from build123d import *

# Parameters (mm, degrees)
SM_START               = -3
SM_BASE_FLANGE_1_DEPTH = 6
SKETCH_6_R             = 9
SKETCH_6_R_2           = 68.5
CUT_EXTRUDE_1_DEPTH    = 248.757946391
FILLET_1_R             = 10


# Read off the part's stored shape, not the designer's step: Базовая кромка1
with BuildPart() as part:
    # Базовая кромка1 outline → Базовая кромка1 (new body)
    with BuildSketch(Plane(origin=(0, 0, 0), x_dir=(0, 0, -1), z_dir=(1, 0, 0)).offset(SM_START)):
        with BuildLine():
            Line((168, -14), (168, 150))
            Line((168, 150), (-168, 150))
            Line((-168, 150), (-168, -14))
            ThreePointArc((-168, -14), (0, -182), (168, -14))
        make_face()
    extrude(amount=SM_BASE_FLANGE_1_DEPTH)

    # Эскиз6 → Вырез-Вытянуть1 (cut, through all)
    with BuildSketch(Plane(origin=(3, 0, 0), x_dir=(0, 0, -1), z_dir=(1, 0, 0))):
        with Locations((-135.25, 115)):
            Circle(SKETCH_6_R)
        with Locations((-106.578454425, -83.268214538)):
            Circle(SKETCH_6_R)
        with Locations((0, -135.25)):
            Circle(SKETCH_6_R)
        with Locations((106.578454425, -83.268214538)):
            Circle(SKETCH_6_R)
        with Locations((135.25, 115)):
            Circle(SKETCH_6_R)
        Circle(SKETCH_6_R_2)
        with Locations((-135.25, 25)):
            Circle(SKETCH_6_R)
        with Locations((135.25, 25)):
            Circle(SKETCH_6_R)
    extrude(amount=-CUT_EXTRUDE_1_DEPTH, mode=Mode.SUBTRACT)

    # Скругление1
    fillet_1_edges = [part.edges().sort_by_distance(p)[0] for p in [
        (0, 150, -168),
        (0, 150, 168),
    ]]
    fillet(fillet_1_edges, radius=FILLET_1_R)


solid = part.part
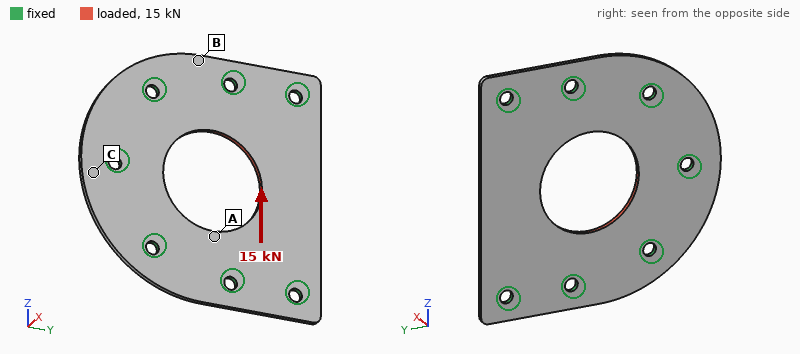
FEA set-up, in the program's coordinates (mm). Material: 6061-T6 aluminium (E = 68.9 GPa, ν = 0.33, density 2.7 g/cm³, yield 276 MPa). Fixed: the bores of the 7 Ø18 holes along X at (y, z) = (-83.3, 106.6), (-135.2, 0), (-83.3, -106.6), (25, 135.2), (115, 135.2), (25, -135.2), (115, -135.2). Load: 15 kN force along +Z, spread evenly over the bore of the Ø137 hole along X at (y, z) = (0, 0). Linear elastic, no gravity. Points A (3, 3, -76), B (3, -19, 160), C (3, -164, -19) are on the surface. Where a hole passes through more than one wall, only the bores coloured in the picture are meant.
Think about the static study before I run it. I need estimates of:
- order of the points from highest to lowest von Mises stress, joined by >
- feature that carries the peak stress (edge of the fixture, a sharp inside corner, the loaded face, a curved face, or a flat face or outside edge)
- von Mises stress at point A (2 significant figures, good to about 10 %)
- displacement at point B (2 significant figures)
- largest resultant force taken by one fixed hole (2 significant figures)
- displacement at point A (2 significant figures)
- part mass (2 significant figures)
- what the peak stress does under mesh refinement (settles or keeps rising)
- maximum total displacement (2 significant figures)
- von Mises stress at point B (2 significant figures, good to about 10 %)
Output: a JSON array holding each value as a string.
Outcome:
["A > B > C", "edge of the fixture", "5.5 MPa", "3.4 µm", "2.9 kN", "6.7 µm", "1.3 kg", "keeps rising", "10 µm", "2.5 MPa"]
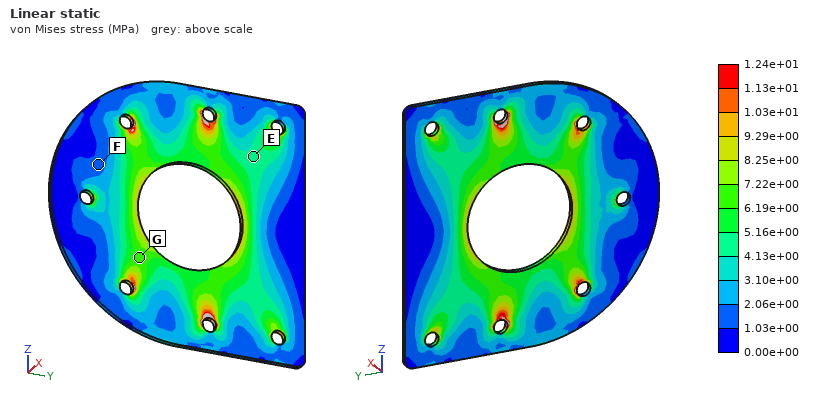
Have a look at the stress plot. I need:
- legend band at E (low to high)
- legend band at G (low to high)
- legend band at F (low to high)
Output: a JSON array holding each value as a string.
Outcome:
["4.13e+00 to 5.16e+00 MPa", "6.19e+00 to 7.22e+00 MPa", "1.03e+00 to 2.06e+00 MPa"]
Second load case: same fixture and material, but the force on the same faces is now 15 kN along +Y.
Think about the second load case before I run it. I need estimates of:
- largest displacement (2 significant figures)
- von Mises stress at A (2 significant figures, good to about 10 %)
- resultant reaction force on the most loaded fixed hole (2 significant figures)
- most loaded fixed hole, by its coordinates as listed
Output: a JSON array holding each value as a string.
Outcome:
["23 µm", "10 MPa", "3.2 kN", "(-135.2, 0)"]
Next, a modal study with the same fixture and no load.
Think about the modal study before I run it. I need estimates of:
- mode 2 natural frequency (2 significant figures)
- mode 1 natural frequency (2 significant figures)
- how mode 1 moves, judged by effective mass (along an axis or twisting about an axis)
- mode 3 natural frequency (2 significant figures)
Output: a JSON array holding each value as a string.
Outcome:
["1100 Hz", "500 Hz", "along X", "1200 Hz"]
